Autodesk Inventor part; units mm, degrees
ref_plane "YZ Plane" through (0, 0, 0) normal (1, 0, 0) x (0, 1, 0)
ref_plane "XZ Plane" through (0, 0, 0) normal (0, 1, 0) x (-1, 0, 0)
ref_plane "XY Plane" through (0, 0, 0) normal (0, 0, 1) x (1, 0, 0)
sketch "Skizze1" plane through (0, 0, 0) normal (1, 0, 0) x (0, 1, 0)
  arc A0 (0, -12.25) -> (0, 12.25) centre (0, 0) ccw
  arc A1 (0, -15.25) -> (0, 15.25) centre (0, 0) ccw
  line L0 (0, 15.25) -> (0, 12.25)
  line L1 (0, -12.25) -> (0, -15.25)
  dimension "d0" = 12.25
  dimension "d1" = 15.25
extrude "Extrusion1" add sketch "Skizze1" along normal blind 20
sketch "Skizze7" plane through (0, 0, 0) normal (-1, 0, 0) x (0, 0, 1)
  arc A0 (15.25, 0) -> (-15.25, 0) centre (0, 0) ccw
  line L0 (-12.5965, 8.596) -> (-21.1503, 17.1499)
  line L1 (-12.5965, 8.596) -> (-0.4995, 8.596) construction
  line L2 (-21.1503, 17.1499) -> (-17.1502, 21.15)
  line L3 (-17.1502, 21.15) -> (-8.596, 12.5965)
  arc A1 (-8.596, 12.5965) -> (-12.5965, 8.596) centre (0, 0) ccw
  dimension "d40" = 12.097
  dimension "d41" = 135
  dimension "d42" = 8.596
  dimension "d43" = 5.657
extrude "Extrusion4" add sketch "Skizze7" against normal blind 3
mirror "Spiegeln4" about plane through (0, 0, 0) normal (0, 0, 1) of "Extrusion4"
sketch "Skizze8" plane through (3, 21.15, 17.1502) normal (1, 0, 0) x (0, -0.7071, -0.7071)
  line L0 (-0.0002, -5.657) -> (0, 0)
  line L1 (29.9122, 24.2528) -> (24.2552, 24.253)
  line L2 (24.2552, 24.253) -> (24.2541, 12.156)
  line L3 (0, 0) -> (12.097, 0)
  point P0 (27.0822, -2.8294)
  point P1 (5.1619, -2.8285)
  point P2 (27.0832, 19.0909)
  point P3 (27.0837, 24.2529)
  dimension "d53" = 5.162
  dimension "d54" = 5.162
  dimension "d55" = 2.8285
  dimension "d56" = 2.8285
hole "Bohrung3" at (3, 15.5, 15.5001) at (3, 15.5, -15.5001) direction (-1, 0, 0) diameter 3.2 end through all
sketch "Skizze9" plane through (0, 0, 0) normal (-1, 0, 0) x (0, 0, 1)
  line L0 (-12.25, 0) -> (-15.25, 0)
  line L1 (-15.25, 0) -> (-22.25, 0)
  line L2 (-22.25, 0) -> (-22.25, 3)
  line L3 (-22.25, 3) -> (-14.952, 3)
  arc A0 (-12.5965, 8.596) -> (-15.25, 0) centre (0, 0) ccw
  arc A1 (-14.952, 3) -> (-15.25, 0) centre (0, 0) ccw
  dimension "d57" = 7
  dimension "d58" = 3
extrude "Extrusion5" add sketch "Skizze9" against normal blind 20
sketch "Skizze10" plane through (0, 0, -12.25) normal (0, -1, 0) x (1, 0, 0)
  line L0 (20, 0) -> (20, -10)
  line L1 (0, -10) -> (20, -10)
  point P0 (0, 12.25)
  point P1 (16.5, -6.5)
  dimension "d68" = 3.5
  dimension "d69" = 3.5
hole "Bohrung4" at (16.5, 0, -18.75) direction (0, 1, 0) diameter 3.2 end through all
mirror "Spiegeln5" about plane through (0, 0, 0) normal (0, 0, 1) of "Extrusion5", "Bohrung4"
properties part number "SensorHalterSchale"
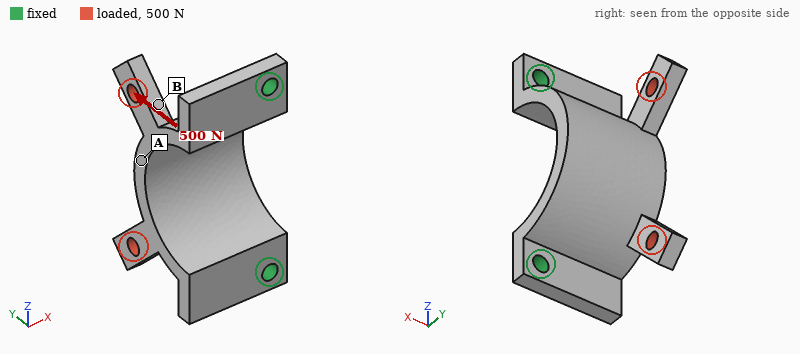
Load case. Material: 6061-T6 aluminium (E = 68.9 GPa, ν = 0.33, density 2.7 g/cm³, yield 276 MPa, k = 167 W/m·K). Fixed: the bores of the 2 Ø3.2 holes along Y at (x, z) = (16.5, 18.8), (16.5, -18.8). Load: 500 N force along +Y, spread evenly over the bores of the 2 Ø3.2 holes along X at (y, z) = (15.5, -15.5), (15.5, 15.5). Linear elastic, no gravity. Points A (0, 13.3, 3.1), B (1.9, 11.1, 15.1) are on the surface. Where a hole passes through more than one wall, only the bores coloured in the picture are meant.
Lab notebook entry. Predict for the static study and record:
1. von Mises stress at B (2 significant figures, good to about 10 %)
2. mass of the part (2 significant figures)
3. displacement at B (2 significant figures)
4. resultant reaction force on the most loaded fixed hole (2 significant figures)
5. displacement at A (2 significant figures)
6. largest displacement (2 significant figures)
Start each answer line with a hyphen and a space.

- 57 MPa
- 10 g
- 0.13 mm
- 260 N
- 0.12 mm
- 0.19 mm
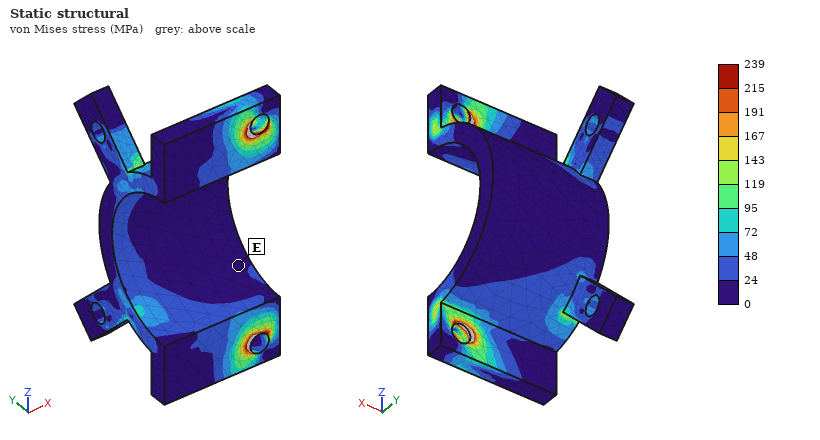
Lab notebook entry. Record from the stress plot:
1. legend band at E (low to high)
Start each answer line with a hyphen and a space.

- 0 to 24 MPa
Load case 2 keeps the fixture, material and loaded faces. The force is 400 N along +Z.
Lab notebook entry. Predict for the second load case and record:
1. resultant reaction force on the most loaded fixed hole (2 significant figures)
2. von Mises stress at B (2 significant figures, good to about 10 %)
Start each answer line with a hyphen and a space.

- 290 N
- 26 MPa
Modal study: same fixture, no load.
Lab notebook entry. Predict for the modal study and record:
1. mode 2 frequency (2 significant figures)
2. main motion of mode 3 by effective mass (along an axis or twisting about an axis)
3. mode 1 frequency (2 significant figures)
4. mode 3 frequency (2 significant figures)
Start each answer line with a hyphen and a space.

- 8200 Hz
- along Z
- 4300 Hz
- 12 kHz
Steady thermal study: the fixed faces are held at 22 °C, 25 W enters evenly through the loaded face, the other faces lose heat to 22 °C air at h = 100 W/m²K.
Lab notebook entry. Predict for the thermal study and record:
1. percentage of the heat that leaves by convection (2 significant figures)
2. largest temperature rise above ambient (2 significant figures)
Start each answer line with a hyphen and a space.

- 23 %
- 66 K
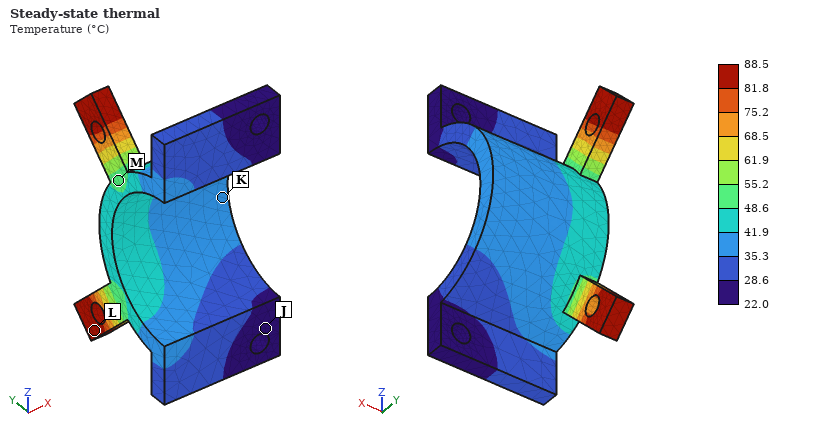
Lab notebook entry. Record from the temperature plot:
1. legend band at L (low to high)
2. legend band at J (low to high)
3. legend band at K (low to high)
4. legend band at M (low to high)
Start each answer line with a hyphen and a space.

- 81.8 to 88.5 °C
- 22.0 to 28.6 °C
- 35.3 to 41.9 °C
- 48.6 to 55.2 °C
